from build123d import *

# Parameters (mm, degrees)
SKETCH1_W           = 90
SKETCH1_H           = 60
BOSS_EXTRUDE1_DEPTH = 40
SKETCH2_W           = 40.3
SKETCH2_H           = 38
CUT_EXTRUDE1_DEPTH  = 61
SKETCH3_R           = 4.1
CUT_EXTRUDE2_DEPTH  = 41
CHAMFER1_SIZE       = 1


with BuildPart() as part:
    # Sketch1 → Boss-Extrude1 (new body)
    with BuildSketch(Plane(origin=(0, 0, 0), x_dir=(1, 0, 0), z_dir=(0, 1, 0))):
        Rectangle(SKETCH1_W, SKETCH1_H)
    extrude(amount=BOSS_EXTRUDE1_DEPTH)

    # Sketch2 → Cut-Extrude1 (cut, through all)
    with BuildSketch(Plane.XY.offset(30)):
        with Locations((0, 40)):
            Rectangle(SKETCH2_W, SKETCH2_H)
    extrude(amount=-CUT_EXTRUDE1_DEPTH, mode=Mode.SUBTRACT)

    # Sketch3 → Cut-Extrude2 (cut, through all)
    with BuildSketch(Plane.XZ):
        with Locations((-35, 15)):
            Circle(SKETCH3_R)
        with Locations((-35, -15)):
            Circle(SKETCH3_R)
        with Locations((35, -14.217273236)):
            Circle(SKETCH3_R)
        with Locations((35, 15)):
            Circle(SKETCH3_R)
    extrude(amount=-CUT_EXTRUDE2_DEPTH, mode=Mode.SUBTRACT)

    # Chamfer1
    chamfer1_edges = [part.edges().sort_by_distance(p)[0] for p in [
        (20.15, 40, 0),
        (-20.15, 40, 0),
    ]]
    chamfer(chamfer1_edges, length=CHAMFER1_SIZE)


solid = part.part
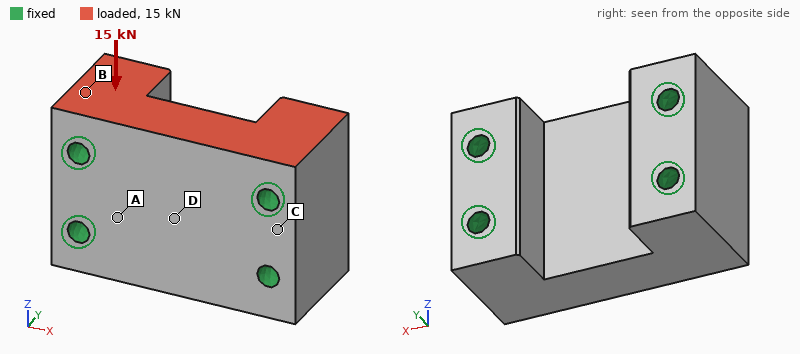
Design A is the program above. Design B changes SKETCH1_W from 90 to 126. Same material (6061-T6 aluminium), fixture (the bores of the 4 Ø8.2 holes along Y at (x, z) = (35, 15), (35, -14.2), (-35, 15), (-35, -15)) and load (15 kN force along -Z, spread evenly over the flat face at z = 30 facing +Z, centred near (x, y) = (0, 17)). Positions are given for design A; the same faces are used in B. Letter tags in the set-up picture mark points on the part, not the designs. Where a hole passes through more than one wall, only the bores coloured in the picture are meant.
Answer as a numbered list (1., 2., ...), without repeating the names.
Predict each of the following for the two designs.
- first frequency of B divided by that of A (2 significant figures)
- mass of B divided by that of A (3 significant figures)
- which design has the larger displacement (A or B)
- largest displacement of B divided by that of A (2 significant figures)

1. 1.00
2. 1.53
3. A
4. 0.69
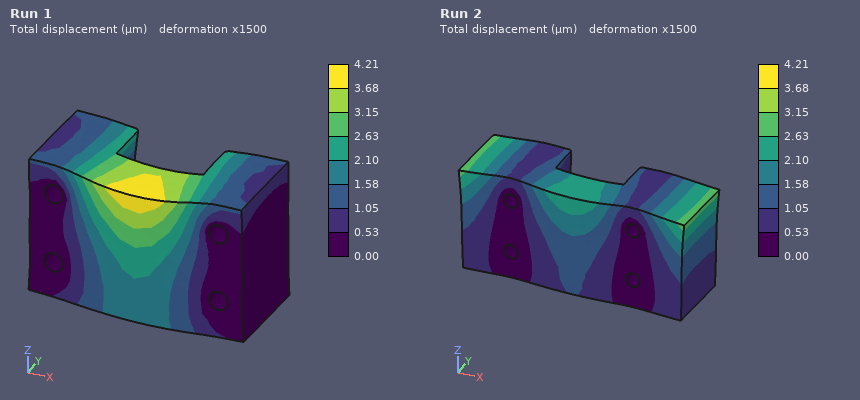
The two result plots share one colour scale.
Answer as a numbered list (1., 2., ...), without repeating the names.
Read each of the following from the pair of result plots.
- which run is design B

1. Run 2
